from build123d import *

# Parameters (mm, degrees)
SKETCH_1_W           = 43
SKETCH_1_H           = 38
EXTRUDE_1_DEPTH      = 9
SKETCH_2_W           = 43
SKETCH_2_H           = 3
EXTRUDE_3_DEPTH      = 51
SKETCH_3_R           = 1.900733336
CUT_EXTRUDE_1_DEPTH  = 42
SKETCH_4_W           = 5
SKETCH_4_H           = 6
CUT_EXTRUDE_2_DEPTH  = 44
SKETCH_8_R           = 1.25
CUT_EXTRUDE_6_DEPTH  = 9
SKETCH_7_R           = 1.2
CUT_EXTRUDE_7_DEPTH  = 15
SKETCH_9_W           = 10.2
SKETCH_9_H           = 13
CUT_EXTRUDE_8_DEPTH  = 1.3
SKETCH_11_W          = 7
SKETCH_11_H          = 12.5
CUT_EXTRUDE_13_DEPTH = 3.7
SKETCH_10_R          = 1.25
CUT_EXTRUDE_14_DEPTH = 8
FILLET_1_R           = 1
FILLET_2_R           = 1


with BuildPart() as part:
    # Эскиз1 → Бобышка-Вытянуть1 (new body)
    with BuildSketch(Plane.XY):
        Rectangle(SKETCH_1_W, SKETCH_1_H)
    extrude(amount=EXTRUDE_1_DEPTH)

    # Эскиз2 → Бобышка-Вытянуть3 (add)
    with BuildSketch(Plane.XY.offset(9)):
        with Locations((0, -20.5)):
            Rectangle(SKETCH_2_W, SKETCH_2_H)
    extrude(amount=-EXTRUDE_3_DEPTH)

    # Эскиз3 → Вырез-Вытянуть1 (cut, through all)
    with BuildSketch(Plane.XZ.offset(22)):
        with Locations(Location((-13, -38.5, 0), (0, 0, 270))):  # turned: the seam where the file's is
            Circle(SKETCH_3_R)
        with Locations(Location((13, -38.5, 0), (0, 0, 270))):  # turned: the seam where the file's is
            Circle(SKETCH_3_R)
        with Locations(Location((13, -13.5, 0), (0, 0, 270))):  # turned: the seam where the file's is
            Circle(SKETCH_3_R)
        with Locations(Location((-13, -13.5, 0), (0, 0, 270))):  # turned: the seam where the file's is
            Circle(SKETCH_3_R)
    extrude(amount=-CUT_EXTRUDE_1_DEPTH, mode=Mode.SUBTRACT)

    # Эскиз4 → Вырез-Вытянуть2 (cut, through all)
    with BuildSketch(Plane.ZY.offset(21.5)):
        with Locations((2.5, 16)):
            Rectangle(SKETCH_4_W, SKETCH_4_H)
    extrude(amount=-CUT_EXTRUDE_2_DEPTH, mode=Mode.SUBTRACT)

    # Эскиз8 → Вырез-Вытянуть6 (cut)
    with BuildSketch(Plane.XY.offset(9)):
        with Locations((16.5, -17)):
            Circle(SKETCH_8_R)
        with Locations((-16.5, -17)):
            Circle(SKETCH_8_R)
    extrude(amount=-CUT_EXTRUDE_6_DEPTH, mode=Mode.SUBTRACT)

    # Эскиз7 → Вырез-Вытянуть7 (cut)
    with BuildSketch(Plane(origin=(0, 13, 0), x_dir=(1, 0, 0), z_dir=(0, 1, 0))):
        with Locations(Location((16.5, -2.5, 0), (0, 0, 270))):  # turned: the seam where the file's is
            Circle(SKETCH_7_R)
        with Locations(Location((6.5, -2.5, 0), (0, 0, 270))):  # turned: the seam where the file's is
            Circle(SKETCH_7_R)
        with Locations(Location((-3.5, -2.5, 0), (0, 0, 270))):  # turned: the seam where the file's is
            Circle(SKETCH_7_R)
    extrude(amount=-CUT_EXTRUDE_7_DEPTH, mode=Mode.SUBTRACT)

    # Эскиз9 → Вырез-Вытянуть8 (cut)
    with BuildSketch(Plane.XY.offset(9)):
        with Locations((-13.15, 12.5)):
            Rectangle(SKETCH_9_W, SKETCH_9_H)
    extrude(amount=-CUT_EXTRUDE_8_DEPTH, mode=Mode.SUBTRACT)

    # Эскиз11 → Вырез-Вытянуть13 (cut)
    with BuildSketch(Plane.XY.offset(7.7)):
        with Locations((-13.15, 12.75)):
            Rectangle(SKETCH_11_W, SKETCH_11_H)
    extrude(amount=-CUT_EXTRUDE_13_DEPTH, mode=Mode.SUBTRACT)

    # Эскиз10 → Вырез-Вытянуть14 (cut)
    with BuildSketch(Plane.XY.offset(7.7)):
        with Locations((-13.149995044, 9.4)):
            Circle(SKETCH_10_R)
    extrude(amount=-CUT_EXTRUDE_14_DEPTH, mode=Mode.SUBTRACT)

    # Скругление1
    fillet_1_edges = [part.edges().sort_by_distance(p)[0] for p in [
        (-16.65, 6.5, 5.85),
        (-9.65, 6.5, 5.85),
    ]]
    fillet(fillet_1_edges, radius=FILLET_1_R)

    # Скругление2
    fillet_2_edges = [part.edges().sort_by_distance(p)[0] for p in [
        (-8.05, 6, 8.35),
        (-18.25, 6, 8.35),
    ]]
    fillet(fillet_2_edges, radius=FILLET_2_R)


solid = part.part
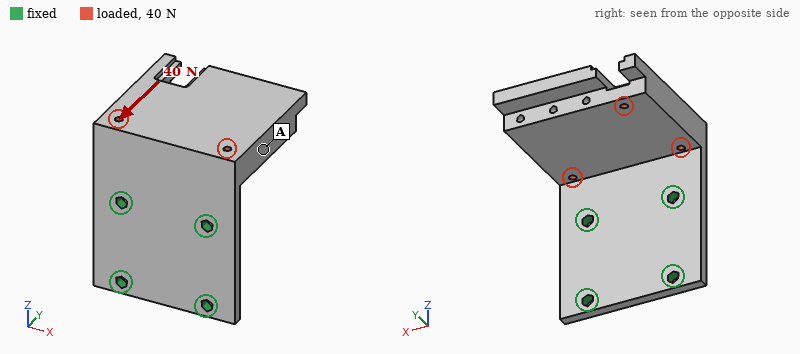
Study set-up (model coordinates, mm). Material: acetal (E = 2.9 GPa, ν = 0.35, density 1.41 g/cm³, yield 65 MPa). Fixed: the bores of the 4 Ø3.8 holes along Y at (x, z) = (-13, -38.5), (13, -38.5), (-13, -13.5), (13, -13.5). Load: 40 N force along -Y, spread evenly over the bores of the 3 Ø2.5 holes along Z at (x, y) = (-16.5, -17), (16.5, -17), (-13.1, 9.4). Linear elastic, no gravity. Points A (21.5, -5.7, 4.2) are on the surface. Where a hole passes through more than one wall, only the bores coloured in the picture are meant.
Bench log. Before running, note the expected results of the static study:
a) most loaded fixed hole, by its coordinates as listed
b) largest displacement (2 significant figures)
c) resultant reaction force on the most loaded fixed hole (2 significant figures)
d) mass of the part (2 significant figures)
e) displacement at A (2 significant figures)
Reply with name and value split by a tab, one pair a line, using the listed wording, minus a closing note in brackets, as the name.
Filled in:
most loaded fixed hole, by its coordinates as listed	(-13, -13.5)
largest displacement	0.86 mm
resultant reaction force on the most loaded fixed hole	26 N
mass of the part	27 g
displacement at A	0.37 mm
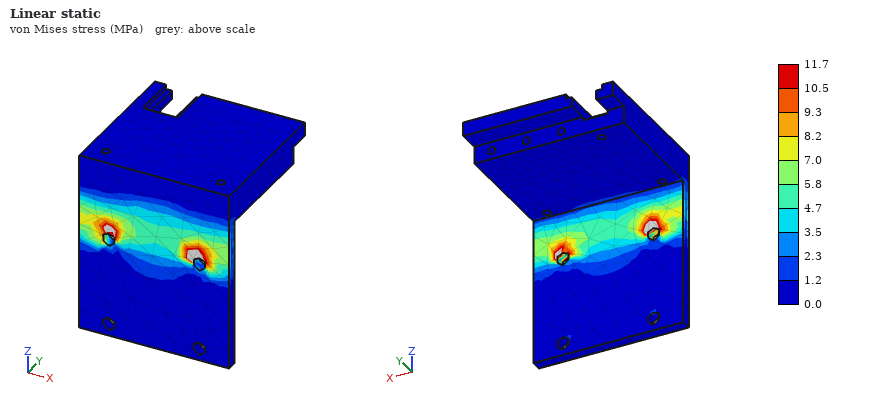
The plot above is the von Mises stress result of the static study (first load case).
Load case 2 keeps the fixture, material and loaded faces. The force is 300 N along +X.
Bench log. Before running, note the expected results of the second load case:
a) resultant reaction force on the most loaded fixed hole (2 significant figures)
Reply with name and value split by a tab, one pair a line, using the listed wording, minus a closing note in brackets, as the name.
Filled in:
resultant reaction force on the most loaded fixed hole	240 N
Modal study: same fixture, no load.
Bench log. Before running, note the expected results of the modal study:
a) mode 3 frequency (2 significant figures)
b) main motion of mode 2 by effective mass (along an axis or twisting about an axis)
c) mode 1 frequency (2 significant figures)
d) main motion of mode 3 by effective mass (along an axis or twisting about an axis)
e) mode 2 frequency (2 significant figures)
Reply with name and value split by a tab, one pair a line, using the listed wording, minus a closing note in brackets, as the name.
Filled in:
mode 3 frequency	1200 Hz
main motion of mode 2 by effective mass	along X
mode 1 frequency	220 Hz
main motion of mode 3 by effective mass	along Y
mode 2 frequency	590 Hz
